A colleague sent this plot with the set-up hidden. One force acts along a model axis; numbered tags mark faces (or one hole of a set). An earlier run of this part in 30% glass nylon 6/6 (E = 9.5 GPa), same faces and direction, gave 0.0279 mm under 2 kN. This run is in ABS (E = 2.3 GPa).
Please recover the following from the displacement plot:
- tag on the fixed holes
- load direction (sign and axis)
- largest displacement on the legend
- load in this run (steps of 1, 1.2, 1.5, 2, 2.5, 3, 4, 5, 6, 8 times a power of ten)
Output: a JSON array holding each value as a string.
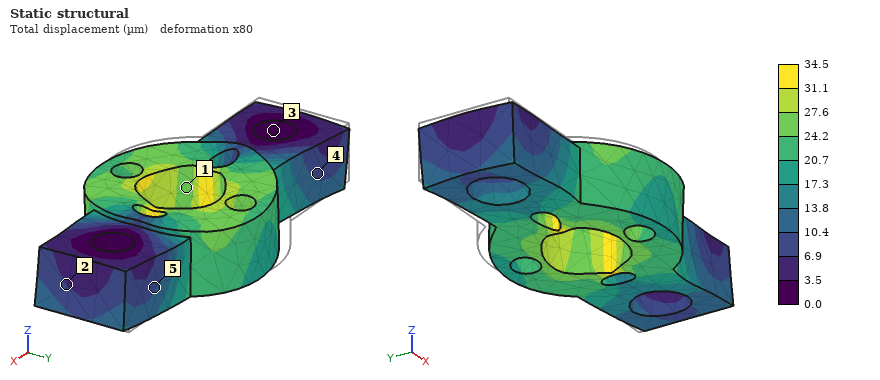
["3", "+X", "34.5 µm", "600 N"]
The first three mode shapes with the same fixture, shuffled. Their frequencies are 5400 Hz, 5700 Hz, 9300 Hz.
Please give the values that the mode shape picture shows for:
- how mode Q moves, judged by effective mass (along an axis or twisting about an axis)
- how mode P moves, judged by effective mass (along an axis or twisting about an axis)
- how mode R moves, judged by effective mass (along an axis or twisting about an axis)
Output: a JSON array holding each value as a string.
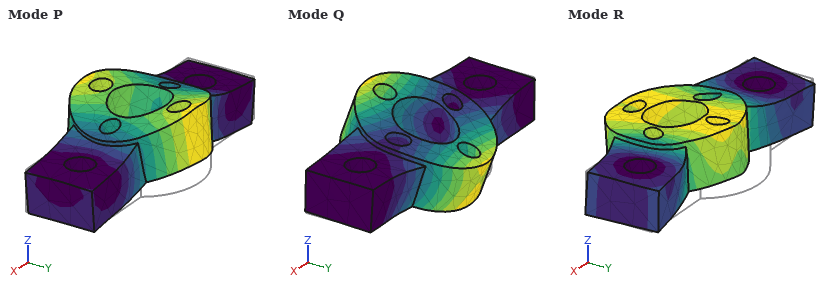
["twisting about X", "along Z", "along Y"]
